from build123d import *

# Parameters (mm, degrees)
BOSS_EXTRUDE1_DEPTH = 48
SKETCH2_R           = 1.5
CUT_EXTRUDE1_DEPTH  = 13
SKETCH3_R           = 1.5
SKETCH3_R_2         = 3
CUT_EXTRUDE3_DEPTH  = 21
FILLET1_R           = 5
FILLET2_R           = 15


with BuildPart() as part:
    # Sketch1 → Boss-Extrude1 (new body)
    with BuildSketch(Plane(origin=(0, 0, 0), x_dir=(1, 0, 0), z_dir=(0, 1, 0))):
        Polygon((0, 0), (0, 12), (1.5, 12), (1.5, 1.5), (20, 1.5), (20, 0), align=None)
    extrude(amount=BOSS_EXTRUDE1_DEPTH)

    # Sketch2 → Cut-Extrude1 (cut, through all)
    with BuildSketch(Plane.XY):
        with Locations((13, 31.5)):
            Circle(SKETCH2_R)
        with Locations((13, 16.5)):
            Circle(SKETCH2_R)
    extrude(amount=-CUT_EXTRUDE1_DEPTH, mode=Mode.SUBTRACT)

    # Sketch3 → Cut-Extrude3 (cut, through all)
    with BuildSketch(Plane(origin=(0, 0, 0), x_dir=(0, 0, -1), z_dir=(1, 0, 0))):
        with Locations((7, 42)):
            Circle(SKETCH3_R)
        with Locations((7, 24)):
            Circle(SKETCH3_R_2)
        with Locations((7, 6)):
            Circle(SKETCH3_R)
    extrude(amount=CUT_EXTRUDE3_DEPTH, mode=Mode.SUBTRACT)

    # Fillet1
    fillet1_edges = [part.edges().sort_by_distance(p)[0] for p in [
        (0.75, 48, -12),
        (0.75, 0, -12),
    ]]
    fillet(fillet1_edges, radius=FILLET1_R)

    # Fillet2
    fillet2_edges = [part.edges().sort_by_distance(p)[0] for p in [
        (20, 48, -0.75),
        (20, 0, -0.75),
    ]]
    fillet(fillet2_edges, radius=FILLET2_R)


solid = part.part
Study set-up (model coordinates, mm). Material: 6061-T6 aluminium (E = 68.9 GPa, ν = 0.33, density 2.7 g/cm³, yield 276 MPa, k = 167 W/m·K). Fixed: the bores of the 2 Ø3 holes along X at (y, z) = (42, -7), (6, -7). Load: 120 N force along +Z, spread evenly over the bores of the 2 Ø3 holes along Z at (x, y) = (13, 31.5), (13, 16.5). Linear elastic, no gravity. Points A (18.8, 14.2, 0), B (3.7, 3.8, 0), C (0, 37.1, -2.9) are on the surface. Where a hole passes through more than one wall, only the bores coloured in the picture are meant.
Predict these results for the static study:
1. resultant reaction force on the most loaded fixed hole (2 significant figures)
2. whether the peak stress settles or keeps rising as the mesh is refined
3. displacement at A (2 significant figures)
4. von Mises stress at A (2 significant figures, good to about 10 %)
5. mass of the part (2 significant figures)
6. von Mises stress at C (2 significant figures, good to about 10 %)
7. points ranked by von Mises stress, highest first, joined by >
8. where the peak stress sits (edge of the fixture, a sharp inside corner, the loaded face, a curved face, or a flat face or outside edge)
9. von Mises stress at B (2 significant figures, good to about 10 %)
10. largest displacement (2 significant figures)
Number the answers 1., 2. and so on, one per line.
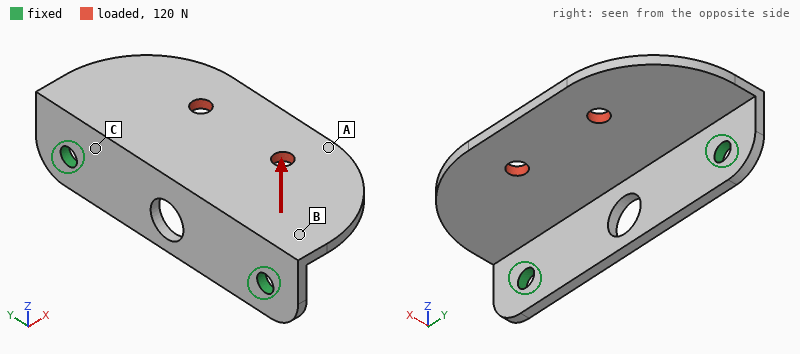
1. 66 N
2. keeps rising
3. 0.37 mm
4. 18 MPa
5. 5.3 g
6. 83 MPa
7. C > B > A
8. edge of the fixture
9. 59 MPa
10. 0.42 mm
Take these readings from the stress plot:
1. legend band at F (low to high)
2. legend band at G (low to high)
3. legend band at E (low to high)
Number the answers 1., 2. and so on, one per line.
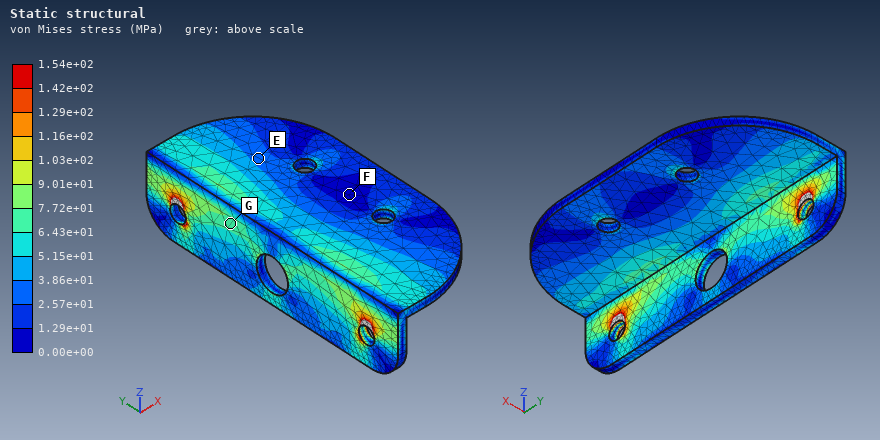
1. 0.00e+00 to 1.29e+01 MPa
2. 6.43e+01 to 7.72e+01 MPa
3. 2.57e+01 to 3.86e+01 MPa
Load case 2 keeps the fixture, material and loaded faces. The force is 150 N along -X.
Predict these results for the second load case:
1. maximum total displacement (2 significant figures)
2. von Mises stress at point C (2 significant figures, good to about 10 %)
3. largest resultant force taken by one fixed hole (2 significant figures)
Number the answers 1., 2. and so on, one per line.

1. 78 µm
2. 19 MPa
3. 78 N
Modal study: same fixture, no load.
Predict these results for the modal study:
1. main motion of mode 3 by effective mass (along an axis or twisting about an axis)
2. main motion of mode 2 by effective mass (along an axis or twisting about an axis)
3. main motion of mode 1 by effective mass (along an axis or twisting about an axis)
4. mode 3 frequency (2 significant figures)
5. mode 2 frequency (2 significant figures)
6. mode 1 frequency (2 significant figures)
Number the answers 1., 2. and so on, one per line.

1. along X
2. twisting about X
3. along Z
4. 7900 Hz
5. 4600 Hz
6. 2300 Hz
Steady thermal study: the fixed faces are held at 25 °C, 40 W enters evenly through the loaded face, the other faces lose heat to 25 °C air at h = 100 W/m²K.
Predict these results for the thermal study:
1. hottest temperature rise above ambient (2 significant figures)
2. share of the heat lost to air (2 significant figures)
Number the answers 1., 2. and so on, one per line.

1. 86 K
2. 28 %
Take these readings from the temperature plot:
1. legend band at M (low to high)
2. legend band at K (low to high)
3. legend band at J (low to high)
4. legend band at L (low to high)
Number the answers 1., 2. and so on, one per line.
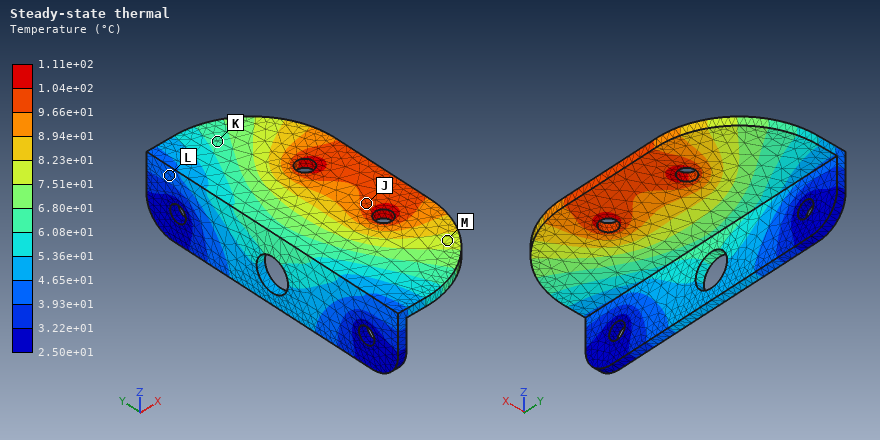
1. 7.51e+01 to 8.23e+01 °C
2. 6.08e+01 to 6.80e+01 °C
3. 9.66e+01 to 1.04e+02 °C
4. 3.93e+01 to 4.65e+01 °C
